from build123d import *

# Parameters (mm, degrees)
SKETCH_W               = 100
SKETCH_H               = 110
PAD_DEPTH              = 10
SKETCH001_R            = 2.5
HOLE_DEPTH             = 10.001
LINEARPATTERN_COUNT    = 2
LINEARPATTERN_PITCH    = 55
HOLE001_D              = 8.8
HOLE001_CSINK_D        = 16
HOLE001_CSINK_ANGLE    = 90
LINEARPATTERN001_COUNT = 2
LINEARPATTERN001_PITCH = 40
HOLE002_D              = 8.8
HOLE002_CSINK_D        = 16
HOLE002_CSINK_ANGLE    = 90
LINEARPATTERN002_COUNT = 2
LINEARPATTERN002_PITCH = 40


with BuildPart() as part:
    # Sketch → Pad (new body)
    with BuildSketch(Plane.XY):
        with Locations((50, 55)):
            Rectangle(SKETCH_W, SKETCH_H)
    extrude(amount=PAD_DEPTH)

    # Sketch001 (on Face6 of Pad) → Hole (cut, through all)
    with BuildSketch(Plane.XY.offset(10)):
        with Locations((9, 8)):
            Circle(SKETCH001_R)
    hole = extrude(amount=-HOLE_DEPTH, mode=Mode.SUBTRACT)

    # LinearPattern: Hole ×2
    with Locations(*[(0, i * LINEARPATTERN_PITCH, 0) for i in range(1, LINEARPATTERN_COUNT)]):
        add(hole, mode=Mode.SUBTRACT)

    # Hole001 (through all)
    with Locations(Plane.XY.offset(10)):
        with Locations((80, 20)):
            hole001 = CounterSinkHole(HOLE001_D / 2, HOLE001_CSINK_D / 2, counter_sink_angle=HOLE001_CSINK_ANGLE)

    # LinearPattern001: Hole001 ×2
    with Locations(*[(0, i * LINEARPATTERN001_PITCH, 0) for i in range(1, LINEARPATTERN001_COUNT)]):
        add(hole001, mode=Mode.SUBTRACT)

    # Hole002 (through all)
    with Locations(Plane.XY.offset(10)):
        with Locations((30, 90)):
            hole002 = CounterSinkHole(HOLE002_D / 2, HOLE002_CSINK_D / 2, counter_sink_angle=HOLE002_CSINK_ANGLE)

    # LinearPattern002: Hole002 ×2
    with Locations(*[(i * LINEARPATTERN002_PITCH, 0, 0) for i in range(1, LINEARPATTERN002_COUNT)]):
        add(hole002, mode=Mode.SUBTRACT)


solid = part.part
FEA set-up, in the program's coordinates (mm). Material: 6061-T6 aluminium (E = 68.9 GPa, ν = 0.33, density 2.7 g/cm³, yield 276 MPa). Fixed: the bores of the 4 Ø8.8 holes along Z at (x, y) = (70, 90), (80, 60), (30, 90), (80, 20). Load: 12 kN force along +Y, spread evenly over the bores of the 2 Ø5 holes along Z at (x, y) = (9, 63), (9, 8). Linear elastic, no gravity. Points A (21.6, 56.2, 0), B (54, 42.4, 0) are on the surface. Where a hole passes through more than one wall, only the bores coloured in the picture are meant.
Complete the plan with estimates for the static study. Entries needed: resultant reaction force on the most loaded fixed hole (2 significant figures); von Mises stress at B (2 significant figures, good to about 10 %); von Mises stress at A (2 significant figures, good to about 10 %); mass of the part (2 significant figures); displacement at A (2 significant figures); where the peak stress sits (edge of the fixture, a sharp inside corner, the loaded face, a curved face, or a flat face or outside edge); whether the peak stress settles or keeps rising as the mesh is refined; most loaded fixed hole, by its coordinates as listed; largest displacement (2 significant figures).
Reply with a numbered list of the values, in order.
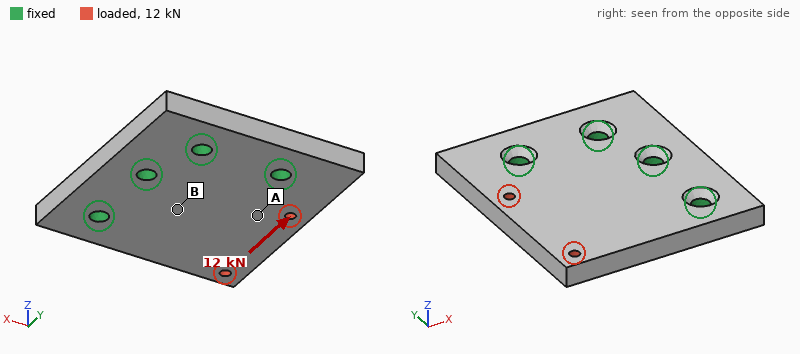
1. 9.9 kN
2. 11 MPa
3. 28 MPa
4. 290 g
5. 19 µm
6. edge of the fixture
7. keeps rising
8. (30, 90)
9. 47 µm
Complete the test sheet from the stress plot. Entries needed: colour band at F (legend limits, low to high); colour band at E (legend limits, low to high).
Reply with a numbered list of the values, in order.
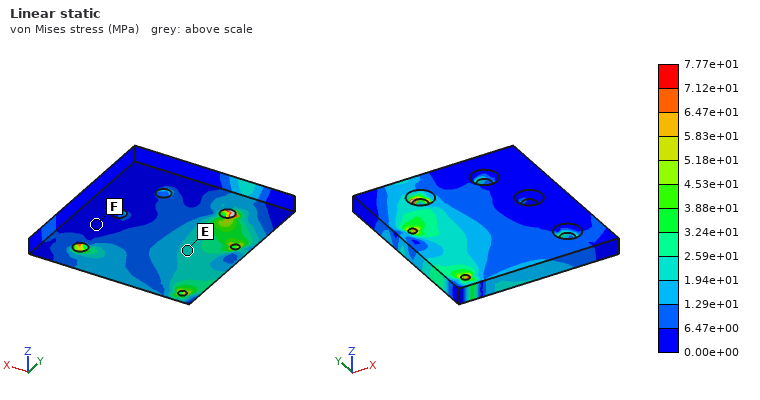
1. 0.00e+00 to 6.47e+00 MPa
2. 1.94e+01 to 2.59e+01 MPa
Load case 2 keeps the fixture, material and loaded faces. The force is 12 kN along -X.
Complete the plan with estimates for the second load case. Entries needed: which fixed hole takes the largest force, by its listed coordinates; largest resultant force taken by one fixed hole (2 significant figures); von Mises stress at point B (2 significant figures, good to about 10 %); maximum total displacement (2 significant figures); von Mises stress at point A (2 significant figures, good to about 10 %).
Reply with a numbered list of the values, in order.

1. (80, 20)
2. 6.7 kN
3. 11 MPa
4. 37 µm
5. 21 MPa
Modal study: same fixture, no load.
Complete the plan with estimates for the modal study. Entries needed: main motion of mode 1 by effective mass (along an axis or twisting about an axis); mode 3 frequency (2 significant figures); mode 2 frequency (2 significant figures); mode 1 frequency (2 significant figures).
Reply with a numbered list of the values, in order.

1. along Z
2. 7700 Hz
3. 5600 Hz
4. 1900 Hz
